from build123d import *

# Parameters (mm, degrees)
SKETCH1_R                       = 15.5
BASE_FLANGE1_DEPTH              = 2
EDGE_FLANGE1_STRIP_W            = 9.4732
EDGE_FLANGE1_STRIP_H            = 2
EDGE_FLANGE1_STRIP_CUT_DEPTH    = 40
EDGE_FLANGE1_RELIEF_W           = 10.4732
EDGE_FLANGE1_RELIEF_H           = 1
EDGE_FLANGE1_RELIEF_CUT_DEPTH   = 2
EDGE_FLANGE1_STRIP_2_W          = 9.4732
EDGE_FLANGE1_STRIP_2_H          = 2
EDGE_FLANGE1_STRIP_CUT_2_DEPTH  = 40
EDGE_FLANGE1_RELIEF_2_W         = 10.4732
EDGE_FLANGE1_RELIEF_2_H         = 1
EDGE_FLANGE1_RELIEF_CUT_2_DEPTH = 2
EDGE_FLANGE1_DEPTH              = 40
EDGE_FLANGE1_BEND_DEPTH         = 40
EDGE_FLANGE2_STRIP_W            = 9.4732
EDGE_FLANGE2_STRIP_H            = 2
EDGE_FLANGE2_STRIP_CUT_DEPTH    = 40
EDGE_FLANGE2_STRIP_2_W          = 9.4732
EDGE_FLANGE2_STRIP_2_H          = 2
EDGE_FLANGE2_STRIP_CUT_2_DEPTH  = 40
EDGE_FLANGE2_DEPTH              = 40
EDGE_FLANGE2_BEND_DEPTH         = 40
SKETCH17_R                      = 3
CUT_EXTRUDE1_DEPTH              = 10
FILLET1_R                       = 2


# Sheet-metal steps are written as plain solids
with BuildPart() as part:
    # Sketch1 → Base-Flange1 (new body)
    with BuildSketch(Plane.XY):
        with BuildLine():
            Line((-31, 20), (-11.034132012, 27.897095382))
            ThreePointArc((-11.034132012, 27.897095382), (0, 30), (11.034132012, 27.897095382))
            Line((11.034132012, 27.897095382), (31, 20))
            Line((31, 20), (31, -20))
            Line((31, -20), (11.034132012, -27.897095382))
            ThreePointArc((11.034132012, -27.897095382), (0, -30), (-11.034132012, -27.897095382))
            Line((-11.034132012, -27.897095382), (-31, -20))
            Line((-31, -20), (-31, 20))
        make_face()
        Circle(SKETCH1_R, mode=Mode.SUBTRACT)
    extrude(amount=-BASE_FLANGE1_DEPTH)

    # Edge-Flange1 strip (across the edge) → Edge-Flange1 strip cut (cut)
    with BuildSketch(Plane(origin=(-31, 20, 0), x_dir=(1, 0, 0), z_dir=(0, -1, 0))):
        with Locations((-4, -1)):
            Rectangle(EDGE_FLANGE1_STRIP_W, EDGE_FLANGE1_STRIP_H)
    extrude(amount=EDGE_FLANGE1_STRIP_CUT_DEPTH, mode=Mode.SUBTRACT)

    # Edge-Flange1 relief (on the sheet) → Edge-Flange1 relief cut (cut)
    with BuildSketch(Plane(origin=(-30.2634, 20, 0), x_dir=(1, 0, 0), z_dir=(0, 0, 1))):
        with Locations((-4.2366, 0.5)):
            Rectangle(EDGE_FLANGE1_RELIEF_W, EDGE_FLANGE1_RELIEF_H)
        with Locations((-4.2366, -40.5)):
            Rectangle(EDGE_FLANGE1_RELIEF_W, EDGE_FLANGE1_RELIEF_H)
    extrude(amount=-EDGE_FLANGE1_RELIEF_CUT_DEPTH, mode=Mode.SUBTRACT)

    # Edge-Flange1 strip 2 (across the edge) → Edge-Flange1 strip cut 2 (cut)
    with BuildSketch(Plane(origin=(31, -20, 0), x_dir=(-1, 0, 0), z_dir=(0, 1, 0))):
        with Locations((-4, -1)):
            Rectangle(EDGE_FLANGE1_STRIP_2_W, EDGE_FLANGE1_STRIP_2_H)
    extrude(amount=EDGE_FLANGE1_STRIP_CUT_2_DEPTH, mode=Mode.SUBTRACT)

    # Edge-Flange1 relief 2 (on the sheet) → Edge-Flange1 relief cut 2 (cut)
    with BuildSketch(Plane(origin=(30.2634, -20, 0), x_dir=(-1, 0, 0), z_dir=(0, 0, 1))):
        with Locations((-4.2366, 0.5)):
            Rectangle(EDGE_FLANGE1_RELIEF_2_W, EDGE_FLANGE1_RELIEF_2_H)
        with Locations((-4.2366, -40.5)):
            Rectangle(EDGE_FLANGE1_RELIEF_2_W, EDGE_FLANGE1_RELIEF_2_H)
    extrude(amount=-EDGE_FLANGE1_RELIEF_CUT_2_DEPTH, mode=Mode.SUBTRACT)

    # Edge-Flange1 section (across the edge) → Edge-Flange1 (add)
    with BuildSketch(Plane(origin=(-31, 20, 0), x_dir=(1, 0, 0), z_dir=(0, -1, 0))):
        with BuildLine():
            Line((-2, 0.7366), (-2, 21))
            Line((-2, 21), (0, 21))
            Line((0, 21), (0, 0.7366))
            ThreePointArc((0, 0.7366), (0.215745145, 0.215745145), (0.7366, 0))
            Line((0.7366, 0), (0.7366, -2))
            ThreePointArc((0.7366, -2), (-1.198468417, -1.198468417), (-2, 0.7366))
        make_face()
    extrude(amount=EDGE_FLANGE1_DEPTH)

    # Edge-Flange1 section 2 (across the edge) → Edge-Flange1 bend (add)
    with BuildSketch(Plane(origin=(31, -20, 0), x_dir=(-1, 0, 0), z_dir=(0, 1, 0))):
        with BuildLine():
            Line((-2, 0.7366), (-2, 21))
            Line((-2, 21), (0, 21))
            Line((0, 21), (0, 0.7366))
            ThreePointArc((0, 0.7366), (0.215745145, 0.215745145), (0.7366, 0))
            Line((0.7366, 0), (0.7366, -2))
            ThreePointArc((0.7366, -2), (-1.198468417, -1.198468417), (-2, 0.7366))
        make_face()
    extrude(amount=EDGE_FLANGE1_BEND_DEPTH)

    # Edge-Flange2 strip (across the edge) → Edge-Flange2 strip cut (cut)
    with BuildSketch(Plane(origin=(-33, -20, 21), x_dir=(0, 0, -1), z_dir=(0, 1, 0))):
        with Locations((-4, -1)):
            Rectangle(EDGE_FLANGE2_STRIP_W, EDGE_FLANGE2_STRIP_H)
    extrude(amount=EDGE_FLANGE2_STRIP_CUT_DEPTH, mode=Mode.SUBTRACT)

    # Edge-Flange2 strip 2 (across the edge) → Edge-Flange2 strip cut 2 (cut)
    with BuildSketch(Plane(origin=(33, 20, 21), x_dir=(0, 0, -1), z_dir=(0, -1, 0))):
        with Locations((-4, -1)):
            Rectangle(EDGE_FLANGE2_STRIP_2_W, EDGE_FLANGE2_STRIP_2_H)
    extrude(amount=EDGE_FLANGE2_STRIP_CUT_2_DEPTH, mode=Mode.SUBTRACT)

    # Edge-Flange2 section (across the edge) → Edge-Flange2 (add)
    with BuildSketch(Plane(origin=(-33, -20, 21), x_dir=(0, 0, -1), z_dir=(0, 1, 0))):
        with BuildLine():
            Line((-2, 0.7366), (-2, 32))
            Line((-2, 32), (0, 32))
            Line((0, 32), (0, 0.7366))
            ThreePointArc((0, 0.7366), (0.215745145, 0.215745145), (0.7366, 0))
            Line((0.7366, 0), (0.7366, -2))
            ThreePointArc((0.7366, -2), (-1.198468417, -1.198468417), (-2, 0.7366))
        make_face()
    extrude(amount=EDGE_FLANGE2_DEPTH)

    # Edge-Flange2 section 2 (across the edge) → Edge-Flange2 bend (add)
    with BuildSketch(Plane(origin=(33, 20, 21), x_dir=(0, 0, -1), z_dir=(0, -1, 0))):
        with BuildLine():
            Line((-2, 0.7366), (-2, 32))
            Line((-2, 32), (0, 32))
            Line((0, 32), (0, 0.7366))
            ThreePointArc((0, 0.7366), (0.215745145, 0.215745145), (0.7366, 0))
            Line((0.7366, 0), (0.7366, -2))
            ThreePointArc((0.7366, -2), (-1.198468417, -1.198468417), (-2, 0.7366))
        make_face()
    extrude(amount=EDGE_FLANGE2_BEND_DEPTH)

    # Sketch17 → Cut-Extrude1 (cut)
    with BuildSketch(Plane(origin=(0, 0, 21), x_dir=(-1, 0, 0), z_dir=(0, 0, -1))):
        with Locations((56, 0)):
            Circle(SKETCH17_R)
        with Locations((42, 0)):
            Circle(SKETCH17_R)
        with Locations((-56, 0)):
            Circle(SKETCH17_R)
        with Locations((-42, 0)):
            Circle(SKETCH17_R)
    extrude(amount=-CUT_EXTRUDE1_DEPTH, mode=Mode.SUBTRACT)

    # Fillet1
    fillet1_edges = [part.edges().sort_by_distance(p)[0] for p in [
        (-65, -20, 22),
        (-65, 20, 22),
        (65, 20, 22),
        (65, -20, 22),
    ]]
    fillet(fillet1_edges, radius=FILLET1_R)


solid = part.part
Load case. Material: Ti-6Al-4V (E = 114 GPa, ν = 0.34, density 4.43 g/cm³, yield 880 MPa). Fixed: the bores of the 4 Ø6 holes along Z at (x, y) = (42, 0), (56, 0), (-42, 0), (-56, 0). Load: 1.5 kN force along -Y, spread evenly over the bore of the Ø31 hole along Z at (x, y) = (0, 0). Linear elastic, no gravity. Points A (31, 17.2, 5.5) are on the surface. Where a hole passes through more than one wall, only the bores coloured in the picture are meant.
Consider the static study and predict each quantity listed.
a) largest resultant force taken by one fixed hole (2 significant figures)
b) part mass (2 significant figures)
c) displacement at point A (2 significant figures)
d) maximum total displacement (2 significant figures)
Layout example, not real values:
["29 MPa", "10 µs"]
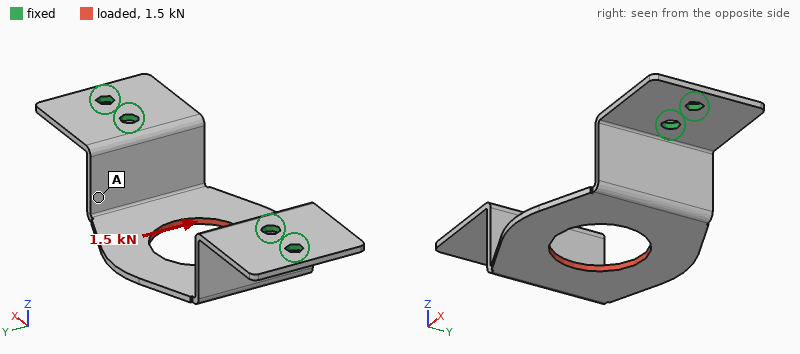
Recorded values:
["1.2 kN", "60 g", "0.55 mm", "0.85 mm"]
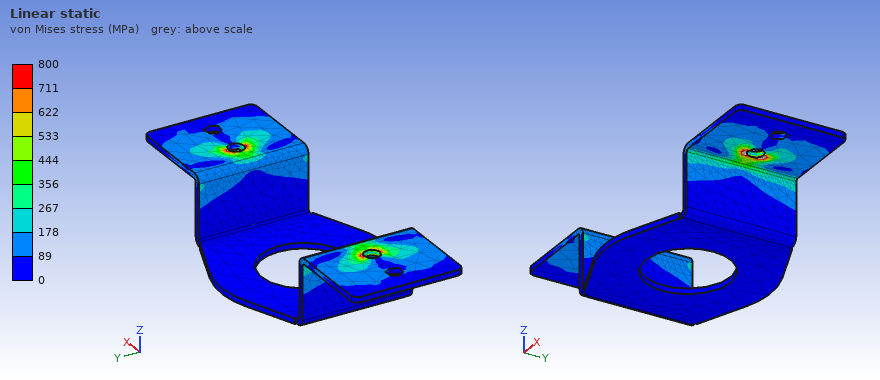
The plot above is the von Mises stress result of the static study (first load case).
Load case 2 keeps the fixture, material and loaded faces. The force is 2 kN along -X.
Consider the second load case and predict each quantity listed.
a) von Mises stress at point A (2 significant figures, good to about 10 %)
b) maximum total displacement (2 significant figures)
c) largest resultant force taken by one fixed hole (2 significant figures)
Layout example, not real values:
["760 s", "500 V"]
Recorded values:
["160 MPa", "1.1 mm", "730 N"]
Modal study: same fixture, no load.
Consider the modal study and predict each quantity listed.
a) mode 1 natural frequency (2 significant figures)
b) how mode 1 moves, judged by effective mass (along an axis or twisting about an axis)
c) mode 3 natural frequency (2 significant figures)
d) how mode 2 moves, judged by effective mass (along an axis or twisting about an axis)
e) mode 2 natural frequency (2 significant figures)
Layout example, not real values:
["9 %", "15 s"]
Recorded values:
["1200 Hz", "along Y", "1700 Hz", "along X", "1300 Hz"]
